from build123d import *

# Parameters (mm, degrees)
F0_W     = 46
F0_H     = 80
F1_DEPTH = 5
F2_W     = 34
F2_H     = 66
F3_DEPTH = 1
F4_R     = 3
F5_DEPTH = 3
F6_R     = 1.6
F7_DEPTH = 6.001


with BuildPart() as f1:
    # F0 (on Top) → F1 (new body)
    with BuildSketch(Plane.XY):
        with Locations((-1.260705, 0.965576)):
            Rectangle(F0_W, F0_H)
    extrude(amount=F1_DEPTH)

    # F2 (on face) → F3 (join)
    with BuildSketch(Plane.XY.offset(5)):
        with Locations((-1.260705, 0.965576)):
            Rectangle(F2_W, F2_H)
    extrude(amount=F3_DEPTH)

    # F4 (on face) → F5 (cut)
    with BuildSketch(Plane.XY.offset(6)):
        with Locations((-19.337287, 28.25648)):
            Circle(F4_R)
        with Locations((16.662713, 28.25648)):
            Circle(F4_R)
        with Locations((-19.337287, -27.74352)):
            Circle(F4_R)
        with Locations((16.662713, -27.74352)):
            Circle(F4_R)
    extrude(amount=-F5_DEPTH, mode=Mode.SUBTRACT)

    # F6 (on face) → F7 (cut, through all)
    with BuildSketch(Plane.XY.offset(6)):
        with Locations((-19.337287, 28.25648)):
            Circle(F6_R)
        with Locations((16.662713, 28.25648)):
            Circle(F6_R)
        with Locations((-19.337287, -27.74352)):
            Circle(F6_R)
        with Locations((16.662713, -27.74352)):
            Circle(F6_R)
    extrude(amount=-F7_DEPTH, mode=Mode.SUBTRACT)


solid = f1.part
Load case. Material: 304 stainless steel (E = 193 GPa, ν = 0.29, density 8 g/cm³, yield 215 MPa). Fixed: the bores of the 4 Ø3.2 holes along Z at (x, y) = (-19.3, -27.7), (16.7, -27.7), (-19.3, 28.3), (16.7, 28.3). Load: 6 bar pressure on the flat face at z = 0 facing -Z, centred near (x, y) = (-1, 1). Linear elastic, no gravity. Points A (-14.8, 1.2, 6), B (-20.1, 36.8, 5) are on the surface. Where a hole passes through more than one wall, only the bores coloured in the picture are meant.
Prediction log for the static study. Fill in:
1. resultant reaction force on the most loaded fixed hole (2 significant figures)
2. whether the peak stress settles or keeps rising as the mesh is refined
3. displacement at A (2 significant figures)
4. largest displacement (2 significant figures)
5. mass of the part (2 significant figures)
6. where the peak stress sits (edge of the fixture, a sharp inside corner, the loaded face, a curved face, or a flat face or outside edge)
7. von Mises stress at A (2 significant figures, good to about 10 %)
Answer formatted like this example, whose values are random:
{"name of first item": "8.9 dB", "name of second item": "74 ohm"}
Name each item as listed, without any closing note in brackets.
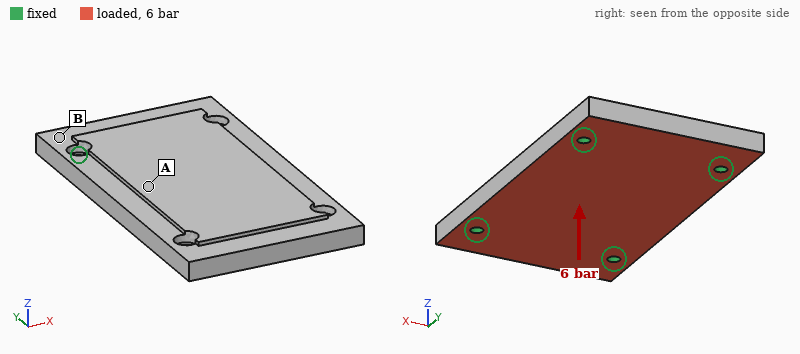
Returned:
{"resultant reaction force on the most loaded fixed hole": "680 N", "whether the peak stress settles or keeps rising as the mesh is refined": "keeps rising", "displacement at A": "11 µm", "largest displacement": "11 µm", "mass of the part": "160 g", "where the peak stress sits": "edge of the fixture", "von Mises stress at A": "23 MPa"}
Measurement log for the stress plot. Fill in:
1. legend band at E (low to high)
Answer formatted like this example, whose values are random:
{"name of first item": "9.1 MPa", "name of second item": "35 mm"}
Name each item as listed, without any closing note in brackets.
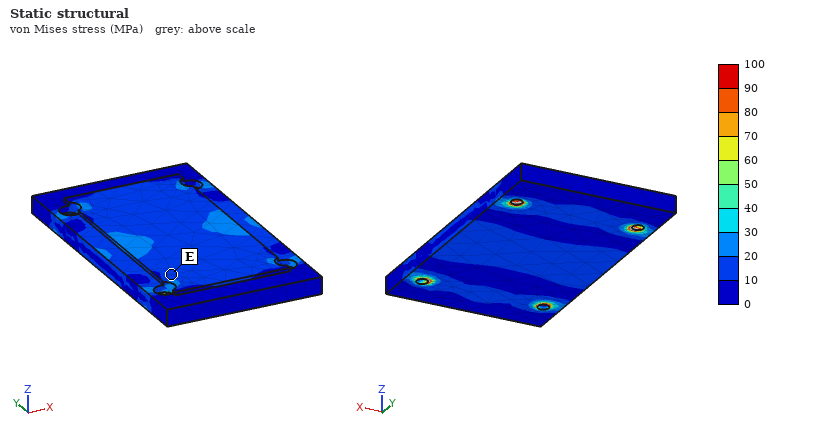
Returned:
{"legend band at E": "10 to 20 MPa"}
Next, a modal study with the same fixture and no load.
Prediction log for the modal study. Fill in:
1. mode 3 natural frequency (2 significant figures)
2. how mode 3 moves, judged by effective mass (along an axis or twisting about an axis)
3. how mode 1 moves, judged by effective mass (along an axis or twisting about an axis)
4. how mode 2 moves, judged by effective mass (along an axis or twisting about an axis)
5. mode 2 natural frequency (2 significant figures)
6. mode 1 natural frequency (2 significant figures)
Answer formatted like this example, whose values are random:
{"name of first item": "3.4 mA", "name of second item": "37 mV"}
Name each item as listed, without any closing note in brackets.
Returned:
{"mode 3 natural frequency": "12 kHz", "how mode 3 moves, judged by effective mass": "along Z", "how mode 1 moves, judged by effective mass": "along Z", "how mode 2 moves, judged by effective mass": "twisting about Y", "mode 2 natural frequency": "9600 Hz", "mode 1 natural frequency": "5900 Hz"}
